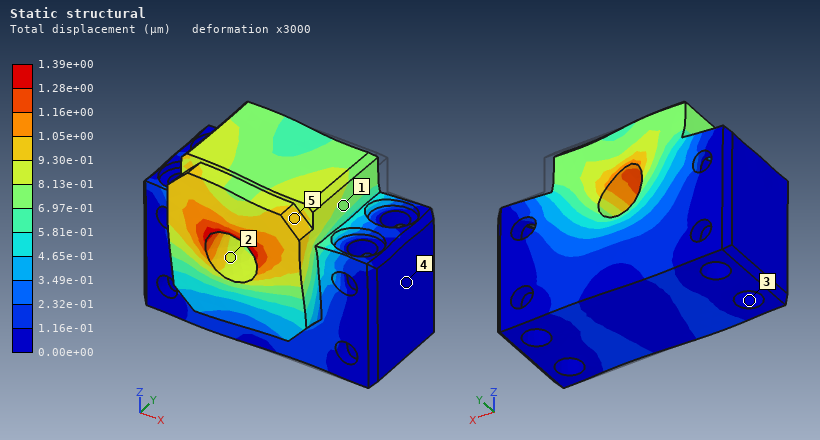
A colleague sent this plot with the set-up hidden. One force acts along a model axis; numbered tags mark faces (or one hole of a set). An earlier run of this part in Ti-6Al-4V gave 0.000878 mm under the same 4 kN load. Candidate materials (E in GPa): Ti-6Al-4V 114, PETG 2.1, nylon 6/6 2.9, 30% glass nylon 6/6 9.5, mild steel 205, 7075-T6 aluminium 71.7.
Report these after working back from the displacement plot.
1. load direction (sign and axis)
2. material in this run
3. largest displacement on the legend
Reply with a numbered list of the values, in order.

1. -X
2. 7075-T6 aluminium
3. 1.39e+00 µm
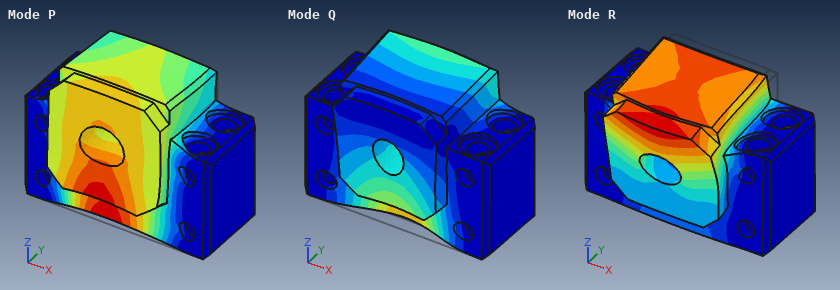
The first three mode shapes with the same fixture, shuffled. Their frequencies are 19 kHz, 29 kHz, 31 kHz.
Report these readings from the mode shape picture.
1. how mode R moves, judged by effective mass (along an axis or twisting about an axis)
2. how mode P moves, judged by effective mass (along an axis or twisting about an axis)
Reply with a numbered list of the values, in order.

1. along Y
2. along Z
